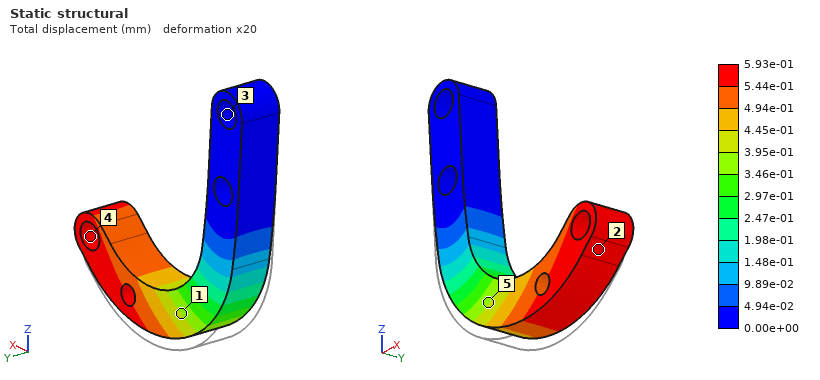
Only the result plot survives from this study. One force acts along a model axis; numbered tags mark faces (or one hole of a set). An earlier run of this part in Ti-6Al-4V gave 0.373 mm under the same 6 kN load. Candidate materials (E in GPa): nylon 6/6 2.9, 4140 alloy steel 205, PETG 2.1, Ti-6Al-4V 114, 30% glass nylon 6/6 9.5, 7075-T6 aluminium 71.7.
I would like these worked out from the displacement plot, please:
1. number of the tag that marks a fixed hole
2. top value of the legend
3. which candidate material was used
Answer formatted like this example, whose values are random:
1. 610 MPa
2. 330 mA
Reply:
1. 3
2. 5.93e-01 mm
3. 7075-T6 aluminium
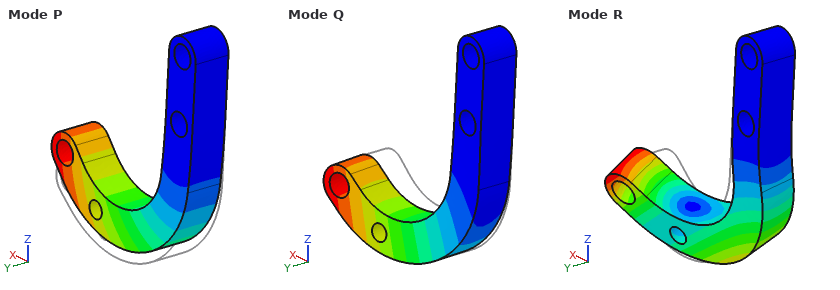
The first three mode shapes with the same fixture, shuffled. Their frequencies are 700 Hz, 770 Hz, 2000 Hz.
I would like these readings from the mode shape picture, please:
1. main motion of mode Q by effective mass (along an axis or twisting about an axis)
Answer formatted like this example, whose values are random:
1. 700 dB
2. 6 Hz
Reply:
1. along Y
